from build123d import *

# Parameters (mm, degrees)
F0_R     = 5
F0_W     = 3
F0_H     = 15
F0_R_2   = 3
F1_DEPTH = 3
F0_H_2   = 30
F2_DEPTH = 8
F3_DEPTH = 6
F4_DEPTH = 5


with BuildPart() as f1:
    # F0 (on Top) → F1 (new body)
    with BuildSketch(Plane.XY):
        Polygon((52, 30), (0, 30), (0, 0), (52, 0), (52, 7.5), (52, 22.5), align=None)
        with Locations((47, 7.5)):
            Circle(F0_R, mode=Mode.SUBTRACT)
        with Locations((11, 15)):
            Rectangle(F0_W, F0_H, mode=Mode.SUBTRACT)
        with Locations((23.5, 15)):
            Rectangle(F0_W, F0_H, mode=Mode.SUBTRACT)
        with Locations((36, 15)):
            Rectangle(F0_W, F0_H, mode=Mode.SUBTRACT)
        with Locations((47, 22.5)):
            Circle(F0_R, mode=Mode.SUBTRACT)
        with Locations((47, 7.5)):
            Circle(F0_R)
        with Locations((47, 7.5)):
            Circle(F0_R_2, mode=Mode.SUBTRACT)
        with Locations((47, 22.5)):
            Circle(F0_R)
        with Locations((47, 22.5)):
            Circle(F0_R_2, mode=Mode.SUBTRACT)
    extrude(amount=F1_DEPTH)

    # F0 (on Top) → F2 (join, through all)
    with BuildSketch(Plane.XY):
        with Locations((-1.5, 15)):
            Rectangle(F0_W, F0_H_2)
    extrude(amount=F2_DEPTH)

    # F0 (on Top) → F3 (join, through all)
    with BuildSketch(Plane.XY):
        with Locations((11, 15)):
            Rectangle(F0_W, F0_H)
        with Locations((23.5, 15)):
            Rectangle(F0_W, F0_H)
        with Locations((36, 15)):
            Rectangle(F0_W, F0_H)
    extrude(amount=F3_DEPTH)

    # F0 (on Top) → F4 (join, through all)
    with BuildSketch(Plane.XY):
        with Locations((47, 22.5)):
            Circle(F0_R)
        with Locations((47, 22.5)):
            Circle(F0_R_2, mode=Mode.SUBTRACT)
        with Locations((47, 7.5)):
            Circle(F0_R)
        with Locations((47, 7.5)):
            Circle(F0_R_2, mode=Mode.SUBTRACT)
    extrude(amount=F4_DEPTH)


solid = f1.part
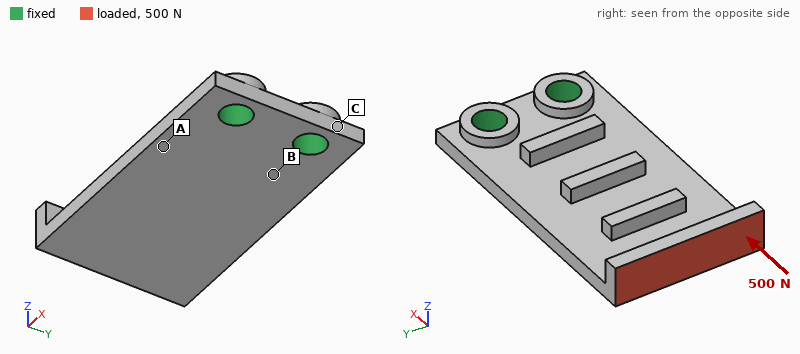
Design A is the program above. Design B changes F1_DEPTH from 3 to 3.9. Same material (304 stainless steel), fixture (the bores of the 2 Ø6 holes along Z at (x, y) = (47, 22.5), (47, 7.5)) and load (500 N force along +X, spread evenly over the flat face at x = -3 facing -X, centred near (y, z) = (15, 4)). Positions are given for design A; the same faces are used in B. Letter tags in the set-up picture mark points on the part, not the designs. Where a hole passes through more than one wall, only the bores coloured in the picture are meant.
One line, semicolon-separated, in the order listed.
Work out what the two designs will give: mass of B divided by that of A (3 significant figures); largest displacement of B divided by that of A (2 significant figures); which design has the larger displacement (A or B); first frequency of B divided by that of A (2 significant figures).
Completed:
1.20; 0.39; A; 1.3
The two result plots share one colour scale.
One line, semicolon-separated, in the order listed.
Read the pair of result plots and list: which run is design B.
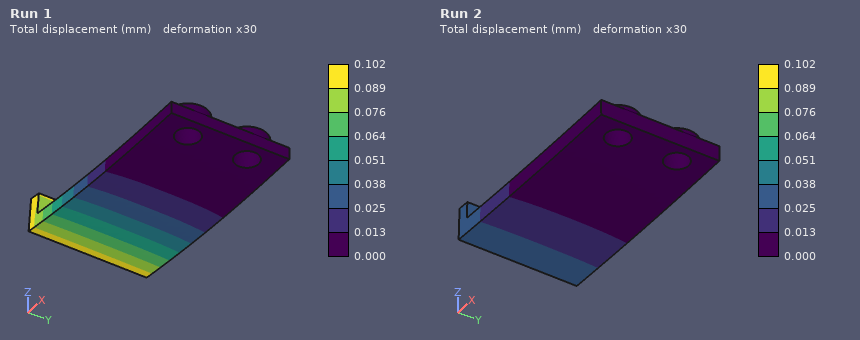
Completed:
Run 2
